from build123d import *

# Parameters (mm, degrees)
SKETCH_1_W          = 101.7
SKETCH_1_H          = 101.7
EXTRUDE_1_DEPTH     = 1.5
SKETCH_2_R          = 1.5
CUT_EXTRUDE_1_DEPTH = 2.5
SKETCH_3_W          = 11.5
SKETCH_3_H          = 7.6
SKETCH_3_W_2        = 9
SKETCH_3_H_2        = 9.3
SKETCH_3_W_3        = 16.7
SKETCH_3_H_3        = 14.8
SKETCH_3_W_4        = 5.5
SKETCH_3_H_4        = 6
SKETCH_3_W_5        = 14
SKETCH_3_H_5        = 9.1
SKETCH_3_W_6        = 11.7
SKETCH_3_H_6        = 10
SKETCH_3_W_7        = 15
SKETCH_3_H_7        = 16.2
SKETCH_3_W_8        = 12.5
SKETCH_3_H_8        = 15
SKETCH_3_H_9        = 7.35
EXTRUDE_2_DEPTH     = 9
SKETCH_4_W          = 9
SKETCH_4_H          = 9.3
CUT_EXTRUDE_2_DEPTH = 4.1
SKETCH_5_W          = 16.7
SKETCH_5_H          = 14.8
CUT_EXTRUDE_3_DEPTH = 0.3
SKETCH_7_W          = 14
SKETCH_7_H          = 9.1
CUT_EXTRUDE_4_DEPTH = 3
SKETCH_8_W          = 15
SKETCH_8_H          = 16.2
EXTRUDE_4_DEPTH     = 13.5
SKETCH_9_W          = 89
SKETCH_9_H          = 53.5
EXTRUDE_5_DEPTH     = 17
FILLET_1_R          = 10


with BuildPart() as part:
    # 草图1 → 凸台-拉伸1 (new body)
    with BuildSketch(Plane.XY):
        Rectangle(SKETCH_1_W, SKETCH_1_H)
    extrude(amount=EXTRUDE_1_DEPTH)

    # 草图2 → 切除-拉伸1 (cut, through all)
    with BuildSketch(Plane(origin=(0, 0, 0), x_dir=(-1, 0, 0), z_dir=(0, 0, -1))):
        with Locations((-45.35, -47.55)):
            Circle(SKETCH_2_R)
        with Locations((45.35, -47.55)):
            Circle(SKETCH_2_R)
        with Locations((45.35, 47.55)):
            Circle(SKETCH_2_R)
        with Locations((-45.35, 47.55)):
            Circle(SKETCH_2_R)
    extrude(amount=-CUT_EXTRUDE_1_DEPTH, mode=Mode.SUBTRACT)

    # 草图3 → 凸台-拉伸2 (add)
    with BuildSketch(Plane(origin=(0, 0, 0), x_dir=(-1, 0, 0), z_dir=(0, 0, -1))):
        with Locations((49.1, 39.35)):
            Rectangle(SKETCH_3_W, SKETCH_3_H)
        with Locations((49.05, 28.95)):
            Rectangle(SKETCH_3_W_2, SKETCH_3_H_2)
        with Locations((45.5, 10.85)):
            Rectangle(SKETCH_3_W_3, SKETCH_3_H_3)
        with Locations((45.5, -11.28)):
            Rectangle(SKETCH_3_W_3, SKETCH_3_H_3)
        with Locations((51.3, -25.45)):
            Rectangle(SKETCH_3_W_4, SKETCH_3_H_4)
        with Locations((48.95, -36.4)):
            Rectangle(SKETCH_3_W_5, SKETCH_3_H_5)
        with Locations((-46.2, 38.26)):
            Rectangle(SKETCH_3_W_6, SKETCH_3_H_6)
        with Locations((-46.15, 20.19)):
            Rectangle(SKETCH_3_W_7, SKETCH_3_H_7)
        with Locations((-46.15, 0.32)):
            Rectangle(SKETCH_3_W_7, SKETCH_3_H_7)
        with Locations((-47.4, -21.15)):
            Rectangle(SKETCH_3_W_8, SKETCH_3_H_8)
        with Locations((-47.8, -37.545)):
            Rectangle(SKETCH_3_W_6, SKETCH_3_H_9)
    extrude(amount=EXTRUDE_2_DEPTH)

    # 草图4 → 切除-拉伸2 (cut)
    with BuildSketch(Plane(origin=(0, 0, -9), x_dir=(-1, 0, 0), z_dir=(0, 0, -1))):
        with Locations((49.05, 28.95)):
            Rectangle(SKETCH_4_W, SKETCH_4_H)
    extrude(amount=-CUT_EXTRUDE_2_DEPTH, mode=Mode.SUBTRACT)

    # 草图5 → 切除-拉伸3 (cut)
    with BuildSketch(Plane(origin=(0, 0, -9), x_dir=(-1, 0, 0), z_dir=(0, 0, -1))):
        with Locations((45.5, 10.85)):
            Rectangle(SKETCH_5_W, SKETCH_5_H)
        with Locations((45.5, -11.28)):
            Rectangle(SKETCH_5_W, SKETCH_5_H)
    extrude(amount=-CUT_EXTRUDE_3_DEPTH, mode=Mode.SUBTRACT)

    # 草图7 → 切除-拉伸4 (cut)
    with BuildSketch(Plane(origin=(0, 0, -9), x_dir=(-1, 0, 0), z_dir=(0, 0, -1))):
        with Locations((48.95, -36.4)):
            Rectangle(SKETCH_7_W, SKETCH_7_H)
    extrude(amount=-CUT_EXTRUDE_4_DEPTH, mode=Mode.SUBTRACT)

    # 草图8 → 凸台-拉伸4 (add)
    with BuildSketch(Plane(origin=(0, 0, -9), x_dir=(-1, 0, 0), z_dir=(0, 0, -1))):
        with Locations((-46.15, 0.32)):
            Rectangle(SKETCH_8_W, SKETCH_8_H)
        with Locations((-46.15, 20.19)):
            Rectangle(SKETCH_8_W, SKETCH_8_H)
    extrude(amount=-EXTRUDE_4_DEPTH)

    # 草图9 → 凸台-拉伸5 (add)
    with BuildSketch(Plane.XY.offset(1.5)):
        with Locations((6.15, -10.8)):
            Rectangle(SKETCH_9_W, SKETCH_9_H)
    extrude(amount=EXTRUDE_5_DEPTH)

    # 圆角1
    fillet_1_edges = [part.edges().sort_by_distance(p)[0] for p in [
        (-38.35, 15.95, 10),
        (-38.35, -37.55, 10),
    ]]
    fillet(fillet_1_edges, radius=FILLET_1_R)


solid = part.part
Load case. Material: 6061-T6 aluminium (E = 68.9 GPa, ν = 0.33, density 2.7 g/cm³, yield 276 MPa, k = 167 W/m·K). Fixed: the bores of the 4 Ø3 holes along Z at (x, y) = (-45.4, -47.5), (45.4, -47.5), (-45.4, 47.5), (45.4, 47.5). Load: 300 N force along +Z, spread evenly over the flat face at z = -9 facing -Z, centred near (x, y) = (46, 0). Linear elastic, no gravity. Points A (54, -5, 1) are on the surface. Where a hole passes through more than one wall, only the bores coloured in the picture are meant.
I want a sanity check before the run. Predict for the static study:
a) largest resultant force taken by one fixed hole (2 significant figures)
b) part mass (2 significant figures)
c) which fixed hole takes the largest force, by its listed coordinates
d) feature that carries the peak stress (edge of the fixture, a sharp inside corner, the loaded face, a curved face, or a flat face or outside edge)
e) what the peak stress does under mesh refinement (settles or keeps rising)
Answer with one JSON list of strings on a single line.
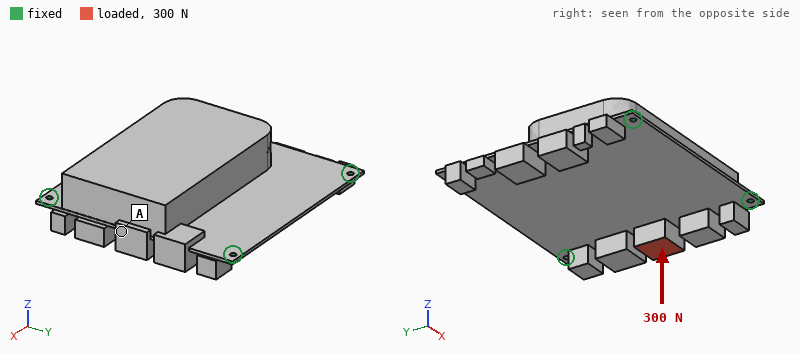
["190 N", "300 g", "(45.4, -47.5)", "edge of the fixture", "keeps rising"]
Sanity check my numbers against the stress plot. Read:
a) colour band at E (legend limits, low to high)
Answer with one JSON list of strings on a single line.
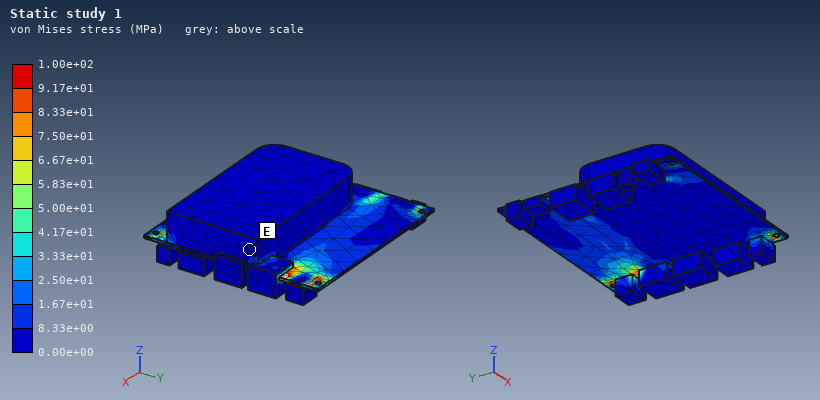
["0.00e+00 to 8.33e+00 MPa"]
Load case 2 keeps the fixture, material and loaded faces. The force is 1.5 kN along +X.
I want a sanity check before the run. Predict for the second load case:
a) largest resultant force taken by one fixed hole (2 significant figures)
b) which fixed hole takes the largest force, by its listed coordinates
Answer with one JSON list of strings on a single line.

["510 N", "(45.4, -47.5)"]
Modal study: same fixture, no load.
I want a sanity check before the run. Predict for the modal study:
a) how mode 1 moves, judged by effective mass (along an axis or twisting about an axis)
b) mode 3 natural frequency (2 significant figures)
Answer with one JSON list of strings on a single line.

["along Z", "1700 Hz"]
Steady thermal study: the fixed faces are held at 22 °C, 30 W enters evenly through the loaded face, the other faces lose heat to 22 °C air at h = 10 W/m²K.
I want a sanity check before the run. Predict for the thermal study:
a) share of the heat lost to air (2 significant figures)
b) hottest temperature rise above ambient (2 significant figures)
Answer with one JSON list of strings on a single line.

["20 %", "37 K"]
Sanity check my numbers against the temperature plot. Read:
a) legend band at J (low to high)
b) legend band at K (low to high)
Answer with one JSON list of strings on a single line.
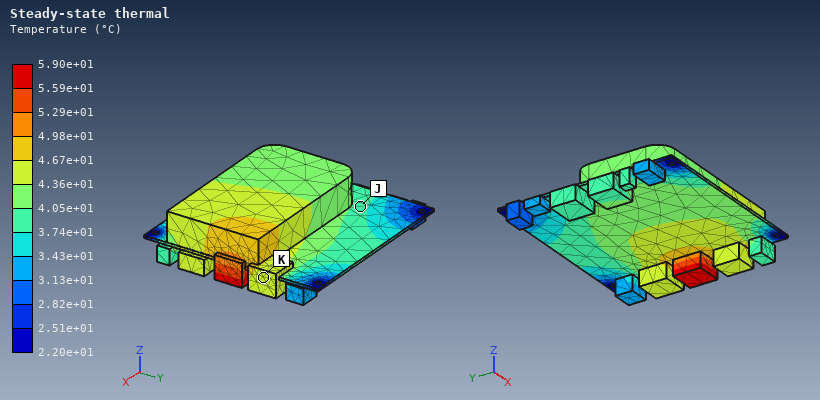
["3.74e+01 to 4.05e+01 °C", "4.36e+01 to 4.67e+01 °C"]
